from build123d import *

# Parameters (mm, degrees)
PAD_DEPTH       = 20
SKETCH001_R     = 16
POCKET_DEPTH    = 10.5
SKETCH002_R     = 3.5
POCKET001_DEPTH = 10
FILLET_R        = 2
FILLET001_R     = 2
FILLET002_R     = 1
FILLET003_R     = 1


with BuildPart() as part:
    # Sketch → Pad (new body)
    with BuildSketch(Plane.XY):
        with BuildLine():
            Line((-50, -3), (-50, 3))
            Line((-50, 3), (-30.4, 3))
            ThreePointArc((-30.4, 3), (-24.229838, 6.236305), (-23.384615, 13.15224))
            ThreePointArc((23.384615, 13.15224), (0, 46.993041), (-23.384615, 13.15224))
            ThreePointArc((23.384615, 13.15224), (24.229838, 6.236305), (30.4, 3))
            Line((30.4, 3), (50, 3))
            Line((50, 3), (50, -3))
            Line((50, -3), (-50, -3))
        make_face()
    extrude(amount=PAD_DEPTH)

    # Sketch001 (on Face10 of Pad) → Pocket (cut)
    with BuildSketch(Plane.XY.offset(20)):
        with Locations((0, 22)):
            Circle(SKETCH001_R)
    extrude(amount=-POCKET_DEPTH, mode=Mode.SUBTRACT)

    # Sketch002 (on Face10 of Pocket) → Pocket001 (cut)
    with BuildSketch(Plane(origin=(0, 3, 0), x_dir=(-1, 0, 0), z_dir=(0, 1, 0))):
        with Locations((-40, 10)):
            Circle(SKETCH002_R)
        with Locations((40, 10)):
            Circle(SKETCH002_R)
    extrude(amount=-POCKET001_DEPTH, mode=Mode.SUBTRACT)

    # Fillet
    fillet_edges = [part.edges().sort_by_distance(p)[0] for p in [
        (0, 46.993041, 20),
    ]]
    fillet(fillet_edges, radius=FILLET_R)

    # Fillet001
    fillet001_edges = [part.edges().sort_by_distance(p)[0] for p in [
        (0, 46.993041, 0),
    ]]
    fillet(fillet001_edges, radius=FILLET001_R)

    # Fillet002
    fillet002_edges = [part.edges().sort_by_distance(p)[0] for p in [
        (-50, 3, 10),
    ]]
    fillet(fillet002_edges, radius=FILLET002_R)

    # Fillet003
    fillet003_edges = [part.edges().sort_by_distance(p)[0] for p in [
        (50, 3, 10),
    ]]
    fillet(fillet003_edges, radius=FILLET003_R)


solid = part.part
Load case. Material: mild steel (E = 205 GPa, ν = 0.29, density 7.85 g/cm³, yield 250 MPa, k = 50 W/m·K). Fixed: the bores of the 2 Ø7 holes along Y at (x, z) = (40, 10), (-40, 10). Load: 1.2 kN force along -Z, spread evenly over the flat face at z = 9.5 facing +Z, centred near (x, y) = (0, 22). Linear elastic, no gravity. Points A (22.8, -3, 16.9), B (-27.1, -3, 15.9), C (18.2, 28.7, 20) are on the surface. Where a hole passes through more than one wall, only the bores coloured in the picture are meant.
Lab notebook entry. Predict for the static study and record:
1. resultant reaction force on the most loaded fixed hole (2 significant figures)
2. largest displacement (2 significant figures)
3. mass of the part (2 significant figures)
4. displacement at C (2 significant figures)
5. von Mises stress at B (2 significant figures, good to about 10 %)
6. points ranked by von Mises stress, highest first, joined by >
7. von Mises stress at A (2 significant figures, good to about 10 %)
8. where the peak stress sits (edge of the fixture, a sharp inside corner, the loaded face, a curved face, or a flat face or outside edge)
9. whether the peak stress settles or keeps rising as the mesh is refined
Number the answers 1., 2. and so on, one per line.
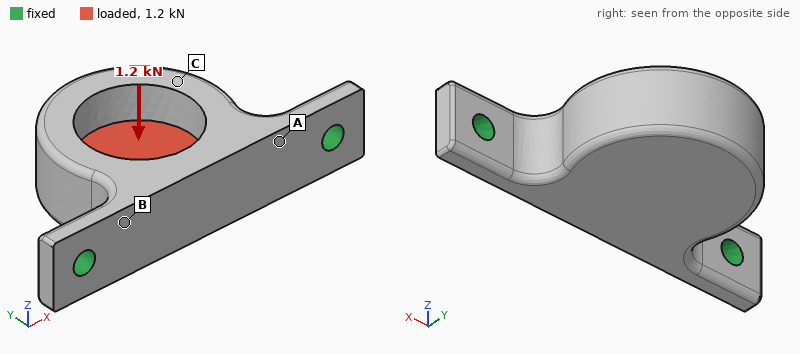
1. 600 N
2. 80 µm
3. 320 g
4. 51 µm
5. 52 MPa
6. B > A > C
7. 40 MPa
8. edge of the fixture
9. keeps rising
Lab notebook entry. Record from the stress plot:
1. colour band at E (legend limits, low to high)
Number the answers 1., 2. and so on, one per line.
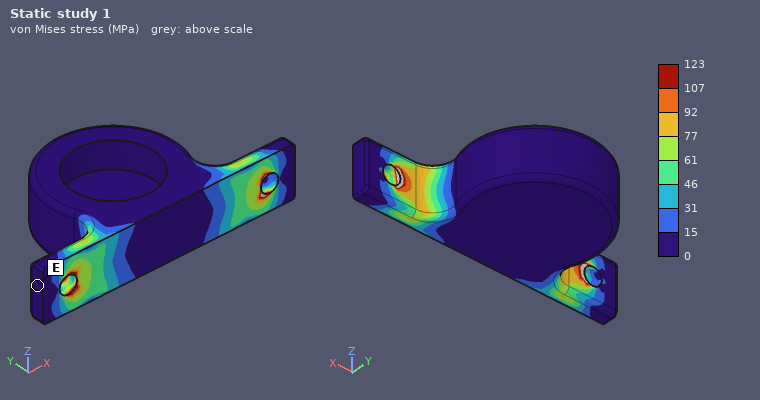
1. 0 to 15 MPa
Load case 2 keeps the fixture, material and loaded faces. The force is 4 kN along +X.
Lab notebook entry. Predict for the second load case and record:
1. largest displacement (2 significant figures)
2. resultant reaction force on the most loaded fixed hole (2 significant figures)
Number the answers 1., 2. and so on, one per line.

1. 16 µm
2. 2.4 kN
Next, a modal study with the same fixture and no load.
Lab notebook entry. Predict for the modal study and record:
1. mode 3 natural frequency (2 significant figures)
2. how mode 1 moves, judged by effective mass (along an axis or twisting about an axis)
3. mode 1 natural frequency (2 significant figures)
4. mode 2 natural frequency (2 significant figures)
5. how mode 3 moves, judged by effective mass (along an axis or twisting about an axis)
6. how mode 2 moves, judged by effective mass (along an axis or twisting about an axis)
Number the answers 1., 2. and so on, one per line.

1. 5700 Hz
2. along Z
3. 1500 Hz
4. 5100 Hz
5. along X
6. along Y
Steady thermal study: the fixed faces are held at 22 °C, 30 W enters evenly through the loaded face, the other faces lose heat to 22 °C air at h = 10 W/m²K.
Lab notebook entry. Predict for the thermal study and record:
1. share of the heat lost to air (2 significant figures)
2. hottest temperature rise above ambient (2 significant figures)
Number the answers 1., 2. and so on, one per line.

1. 13 %
2. 60 K
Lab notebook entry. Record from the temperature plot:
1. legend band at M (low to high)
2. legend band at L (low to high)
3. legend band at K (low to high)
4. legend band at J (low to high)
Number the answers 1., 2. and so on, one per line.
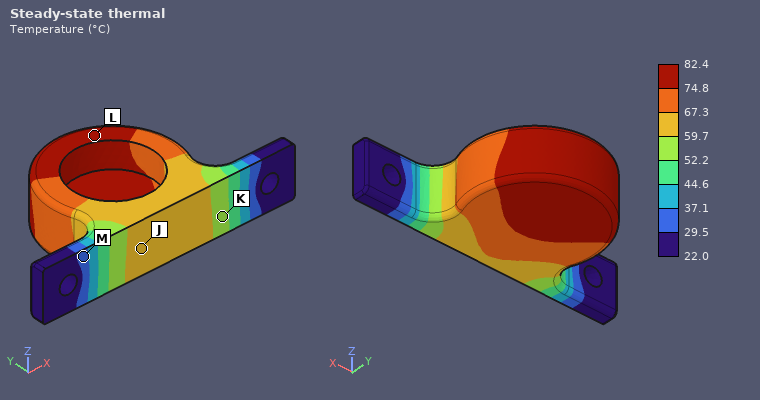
1. 29.5 to 37.1 °C
2. 74.8 to 82.4 °C
3. 52.2 to 59.7 °C
4. 59.7 to 67.3 °C
